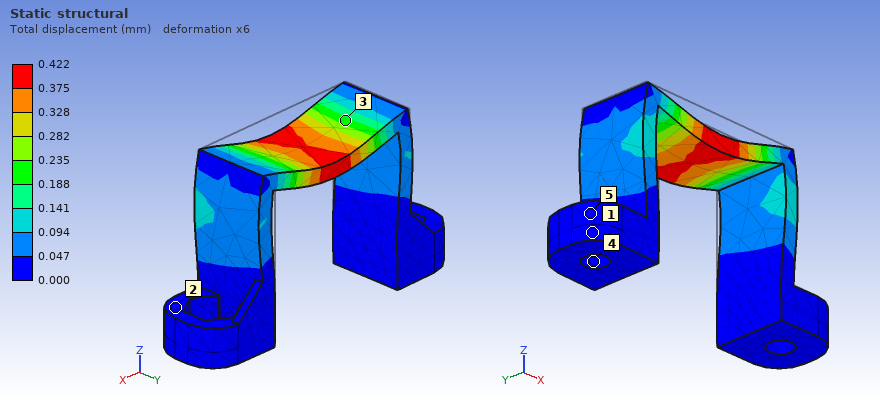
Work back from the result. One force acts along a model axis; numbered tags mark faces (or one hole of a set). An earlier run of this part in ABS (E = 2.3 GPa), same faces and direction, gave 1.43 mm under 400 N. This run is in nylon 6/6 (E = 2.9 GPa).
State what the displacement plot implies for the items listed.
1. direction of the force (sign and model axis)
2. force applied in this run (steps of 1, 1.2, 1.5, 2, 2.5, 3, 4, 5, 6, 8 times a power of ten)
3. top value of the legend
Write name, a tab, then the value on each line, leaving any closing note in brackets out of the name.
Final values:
direction of the force	-Z
force applied in this run	150 N
top value of the legend	0.422 mm
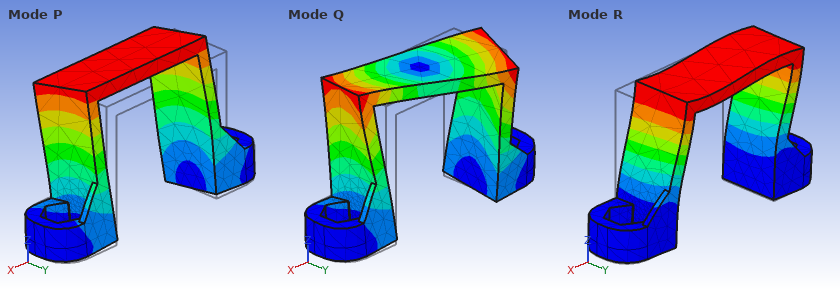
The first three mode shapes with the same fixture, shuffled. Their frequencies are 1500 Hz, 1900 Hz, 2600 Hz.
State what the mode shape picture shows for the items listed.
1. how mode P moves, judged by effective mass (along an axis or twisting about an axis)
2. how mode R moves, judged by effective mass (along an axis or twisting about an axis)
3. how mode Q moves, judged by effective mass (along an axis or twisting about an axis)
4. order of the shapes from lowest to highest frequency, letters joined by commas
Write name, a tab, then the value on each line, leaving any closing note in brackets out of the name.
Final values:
how mode P moves, judged by effective mass	along Y
how mode R moves, judged by effective mass	along X
how mode Q moves, judged by effective mass	twisting about Z
order of the shapes from lowest to highest frequency, letters joined by commas	R, P, Q
